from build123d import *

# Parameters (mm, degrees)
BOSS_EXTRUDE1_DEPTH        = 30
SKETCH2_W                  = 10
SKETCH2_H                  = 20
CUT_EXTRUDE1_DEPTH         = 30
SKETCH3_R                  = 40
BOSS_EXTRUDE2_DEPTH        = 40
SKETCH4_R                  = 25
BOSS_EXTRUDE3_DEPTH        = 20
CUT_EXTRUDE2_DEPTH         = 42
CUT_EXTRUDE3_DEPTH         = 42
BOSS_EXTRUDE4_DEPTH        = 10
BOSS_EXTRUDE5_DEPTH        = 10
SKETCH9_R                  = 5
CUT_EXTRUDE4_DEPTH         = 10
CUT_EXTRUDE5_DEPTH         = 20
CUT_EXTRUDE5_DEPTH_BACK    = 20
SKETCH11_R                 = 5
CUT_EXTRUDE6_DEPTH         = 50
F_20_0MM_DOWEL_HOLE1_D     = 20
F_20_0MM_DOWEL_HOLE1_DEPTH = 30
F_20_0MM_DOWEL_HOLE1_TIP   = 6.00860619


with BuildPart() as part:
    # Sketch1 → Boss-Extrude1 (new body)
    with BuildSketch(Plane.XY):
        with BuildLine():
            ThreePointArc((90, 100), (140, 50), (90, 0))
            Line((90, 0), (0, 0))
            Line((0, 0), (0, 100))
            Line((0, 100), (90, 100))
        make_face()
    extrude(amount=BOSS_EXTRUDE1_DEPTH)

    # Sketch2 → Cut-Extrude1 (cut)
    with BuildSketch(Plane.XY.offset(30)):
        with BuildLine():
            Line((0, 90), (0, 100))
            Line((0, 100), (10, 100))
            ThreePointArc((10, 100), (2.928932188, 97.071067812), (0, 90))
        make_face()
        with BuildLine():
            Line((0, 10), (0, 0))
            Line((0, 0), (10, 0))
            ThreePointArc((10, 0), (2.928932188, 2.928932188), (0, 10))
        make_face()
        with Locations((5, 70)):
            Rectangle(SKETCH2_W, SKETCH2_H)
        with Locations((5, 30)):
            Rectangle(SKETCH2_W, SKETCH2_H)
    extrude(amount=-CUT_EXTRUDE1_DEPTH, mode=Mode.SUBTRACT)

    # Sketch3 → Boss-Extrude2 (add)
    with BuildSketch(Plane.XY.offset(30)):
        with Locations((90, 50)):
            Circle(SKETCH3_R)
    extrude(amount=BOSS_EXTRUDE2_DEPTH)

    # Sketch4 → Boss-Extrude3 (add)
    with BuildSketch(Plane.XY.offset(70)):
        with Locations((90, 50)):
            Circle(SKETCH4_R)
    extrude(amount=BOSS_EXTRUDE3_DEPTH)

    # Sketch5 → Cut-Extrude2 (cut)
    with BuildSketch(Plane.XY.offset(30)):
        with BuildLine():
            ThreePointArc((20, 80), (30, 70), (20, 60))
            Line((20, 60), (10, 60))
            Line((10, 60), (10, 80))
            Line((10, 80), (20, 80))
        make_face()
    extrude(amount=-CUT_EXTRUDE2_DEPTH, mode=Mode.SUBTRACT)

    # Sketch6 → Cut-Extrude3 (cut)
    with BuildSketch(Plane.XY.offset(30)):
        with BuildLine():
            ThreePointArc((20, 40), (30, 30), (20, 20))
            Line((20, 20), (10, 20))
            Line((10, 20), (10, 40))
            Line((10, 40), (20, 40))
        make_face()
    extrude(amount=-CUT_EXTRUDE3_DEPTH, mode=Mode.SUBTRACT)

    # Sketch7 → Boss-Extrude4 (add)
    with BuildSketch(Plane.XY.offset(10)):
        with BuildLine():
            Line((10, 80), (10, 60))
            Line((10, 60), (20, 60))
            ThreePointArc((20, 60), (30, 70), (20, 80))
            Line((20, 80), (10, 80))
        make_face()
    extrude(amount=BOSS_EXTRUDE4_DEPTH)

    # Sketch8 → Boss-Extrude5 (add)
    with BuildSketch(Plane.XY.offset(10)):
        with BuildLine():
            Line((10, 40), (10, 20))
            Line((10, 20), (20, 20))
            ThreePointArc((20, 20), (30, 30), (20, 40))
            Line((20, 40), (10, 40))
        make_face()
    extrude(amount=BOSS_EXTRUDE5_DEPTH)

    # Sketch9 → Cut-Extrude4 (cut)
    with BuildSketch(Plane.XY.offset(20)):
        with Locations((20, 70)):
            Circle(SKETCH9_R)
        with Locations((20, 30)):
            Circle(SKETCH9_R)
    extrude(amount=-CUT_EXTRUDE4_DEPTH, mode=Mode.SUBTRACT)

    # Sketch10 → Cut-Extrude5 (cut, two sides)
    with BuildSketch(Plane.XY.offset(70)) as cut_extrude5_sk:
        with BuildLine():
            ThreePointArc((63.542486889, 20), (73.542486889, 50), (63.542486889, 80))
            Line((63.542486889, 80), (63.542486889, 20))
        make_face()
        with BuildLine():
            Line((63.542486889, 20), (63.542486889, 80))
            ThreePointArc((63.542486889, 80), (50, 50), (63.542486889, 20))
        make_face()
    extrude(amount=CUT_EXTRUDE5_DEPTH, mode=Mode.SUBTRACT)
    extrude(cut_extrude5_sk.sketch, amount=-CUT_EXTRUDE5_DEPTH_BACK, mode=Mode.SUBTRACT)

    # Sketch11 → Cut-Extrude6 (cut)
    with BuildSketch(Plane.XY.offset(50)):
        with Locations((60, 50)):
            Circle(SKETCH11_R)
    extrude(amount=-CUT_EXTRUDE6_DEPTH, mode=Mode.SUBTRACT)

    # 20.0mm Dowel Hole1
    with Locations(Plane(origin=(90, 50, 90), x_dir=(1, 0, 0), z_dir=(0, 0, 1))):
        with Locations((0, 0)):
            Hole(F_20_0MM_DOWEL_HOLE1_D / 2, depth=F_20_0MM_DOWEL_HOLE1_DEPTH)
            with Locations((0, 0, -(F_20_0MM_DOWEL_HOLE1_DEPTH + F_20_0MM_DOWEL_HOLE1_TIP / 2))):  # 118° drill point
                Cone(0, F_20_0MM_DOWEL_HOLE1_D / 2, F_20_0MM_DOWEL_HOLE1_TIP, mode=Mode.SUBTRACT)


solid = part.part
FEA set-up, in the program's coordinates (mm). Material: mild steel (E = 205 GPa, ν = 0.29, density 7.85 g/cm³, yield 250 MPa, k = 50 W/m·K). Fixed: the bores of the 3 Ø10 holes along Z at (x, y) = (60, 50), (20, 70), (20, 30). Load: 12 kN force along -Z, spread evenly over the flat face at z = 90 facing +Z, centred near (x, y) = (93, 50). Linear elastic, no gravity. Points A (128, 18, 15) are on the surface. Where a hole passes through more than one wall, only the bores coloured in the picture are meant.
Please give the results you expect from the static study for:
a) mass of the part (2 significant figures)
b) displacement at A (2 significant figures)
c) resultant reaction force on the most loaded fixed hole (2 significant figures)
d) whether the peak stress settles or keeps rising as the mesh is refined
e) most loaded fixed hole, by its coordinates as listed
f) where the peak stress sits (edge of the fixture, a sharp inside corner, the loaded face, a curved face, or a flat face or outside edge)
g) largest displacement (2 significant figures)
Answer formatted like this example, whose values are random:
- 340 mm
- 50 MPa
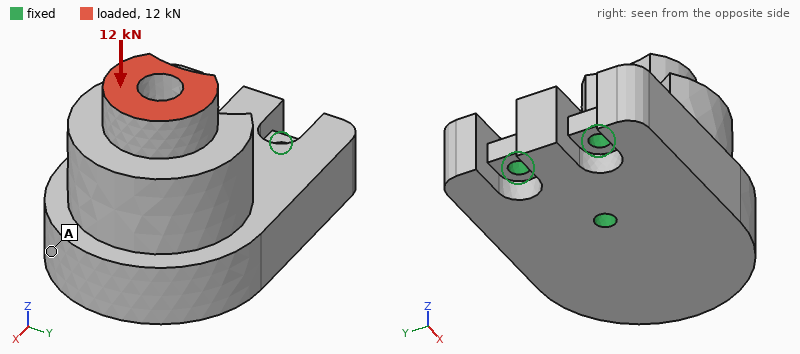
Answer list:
- 4.4 kg
- 7.0 µm
- 13 kN
- keeps rising
- (60, 50)
- edge of the fixture
- 9.5 µm
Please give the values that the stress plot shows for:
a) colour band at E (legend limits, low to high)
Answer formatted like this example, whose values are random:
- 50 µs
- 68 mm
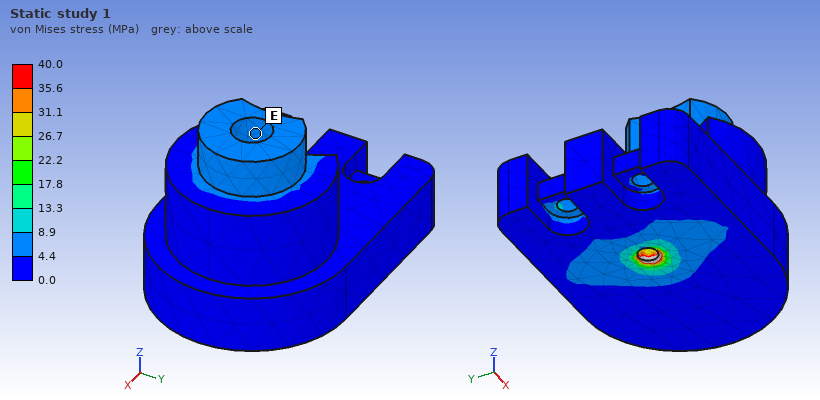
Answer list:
- 4.4 to 8.9 MPa
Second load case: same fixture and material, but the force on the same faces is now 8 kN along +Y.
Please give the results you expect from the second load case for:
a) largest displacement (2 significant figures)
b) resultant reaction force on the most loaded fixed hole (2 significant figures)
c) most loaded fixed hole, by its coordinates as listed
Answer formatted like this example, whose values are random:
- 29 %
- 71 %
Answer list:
- 17 µm
- 11 kN
- (60, 50)
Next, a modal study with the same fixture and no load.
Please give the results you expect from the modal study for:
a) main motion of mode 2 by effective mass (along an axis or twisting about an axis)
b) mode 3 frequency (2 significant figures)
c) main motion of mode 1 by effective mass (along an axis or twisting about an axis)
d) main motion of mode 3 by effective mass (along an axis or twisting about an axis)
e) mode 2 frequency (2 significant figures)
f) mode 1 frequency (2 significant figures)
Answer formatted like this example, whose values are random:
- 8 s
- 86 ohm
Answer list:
- along Y
- 5200 Hz
- along Z
- twisting about X
- 4100 Hz
- 3700 Hz
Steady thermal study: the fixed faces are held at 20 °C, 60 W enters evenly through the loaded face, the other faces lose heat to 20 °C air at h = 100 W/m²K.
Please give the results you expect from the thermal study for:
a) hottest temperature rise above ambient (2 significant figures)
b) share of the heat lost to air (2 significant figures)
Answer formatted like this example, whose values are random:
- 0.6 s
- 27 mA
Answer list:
- 31 K
- 50 %
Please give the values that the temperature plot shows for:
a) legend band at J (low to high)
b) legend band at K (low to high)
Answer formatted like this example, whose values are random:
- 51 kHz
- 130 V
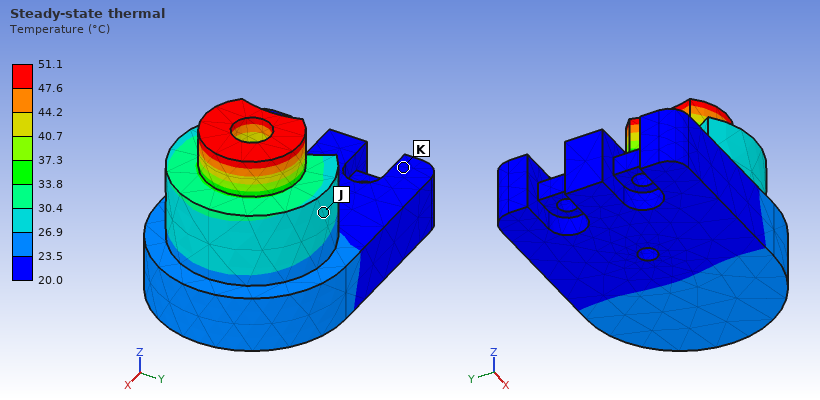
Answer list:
- 26.9 to 30.4 °C
- 20.0 to 23.5 °C
